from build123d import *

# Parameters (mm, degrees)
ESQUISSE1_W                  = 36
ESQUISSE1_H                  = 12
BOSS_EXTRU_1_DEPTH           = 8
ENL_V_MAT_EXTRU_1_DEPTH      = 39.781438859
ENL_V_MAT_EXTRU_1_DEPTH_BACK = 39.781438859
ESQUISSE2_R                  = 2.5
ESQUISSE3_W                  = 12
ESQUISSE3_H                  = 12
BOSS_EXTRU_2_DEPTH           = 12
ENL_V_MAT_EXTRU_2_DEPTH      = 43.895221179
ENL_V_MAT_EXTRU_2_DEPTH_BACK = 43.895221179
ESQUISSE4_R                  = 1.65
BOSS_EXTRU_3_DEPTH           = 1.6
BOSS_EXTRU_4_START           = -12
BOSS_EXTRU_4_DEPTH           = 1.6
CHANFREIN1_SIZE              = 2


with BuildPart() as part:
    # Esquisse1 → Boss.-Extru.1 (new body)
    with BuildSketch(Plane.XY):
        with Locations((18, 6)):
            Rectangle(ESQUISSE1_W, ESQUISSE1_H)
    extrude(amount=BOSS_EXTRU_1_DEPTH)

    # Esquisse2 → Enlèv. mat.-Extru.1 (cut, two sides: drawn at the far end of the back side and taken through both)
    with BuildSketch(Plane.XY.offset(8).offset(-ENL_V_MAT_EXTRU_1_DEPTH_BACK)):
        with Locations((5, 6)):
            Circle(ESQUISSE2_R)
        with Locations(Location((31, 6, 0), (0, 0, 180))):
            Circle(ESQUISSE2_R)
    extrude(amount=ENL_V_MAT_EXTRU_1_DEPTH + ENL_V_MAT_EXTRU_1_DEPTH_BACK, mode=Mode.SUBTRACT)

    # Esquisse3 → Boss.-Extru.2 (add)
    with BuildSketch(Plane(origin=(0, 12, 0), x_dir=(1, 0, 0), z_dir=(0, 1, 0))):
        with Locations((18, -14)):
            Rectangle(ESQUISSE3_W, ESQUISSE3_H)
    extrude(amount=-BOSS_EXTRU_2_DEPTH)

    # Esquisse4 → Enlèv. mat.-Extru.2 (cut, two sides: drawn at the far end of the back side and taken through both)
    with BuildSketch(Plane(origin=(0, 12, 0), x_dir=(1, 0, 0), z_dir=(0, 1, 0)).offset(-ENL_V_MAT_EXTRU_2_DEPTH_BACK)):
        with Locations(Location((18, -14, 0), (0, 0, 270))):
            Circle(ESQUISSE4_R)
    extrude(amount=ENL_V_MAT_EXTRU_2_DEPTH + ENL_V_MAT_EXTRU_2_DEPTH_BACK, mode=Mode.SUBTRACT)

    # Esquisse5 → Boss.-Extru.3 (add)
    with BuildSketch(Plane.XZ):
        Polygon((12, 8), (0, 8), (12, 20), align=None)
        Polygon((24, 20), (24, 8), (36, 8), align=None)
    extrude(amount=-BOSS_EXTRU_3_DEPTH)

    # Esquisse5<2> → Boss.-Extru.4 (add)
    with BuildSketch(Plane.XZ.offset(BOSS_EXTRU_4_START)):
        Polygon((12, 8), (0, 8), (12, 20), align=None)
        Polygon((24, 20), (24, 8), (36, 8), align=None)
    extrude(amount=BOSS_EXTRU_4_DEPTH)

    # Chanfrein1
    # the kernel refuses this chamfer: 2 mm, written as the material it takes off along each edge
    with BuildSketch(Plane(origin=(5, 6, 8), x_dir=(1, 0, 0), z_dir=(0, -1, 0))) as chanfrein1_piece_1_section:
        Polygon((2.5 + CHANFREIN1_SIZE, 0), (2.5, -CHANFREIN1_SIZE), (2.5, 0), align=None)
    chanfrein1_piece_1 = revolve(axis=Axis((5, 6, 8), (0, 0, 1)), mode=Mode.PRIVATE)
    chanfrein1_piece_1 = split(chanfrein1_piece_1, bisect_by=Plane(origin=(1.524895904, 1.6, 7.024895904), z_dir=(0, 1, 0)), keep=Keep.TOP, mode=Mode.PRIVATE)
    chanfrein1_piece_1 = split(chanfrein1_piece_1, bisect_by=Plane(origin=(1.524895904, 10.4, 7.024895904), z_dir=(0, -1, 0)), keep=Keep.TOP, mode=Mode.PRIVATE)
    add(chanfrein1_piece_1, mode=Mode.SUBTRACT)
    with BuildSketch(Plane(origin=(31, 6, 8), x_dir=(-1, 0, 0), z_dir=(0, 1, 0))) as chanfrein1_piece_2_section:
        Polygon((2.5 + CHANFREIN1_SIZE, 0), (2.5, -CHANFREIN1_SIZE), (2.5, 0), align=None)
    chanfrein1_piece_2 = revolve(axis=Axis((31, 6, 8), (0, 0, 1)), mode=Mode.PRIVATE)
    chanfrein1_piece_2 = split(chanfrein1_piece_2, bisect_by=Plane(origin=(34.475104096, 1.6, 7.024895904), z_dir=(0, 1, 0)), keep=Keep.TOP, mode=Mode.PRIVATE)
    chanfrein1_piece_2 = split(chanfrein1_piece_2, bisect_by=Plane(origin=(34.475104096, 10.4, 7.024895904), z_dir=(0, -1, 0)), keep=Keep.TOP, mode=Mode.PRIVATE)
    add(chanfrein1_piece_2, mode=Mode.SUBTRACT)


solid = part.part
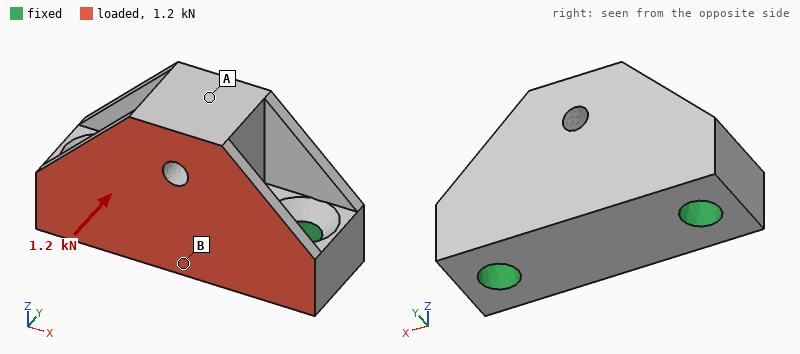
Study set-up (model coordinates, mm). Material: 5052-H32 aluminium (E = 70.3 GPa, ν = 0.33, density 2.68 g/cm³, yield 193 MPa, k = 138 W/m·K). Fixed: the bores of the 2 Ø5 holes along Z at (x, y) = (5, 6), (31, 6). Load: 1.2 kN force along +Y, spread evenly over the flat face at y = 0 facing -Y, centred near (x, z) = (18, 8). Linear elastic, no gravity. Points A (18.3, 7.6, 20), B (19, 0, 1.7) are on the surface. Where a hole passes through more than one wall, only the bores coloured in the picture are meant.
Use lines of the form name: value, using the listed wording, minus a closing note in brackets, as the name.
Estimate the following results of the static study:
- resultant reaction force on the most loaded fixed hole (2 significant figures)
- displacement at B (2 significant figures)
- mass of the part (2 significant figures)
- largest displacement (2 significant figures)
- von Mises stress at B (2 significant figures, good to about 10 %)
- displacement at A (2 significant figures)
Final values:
resultant reaction force on the most loaded fixed hole: 600 N
displacement at B: 3.5 µm
mass of the part: 14 g
largest displacement: 16 µm
von Mises stress at B: 9.4 MPa
displacement at A: 13 µm
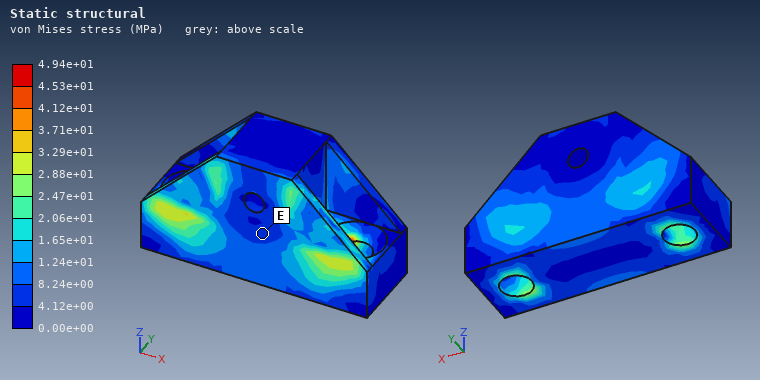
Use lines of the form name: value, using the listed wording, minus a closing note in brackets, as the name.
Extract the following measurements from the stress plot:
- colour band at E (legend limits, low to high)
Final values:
colour band at E: 4.12e+00 to 8.24e+00 MPa
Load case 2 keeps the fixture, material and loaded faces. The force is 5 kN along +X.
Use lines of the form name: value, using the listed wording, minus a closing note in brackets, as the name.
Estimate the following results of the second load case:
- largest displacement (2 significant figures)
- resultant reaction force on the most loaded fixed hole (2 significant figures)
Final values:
largest displacement: 21 µm
resultant reaction force on the most loaded fixed hole: 2.8 kN
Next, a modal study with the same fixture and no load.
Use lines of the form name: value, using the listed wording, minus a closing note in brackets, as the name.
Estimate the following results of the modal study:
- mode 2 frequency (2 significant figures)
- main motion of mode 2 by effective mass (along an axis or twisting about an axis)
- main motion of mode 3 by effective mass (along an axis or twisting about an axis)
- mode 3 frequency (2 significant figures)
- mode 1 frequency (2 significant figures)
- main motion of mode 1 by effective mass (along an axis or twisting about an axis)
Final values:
mode 2 frequency: 37 kHz
main motion of mode 2 by effective mass: along Z
main motion of mode 3 by effective mass: along X
mode 3 frequency: 39 kHz
mode 1 frequency: 16 kHz
main motion of mode 1 by effective mass: along Y
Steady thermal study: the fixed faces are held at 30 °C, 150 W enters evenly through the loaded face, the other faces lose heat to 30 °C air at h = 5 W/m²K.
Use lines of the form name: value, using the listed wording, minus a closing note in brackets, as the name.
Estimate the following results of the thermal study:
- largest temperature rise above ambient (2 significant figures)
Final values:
largest temperature rise above ambient: 58 K
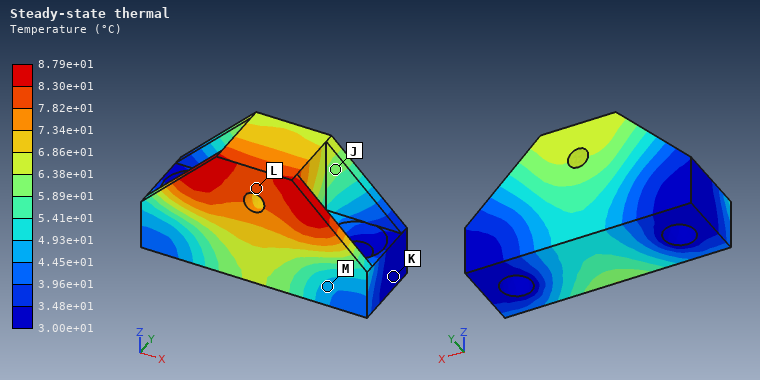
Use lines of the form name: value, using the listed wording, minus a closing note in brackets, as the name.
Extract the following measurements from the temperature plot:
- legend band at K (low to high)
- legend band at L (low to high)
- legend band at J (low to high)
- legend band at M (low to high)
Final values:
legend band at K: 3.00e+01 to 3.48e+01 °C
legend band at L: 7.82e+01 to 8.30e+01 °C
legend band at J: 5.89e+01 to 6.38e+01 °C
legend band at M: 4.45e+01 to 4.93e+01 °C
